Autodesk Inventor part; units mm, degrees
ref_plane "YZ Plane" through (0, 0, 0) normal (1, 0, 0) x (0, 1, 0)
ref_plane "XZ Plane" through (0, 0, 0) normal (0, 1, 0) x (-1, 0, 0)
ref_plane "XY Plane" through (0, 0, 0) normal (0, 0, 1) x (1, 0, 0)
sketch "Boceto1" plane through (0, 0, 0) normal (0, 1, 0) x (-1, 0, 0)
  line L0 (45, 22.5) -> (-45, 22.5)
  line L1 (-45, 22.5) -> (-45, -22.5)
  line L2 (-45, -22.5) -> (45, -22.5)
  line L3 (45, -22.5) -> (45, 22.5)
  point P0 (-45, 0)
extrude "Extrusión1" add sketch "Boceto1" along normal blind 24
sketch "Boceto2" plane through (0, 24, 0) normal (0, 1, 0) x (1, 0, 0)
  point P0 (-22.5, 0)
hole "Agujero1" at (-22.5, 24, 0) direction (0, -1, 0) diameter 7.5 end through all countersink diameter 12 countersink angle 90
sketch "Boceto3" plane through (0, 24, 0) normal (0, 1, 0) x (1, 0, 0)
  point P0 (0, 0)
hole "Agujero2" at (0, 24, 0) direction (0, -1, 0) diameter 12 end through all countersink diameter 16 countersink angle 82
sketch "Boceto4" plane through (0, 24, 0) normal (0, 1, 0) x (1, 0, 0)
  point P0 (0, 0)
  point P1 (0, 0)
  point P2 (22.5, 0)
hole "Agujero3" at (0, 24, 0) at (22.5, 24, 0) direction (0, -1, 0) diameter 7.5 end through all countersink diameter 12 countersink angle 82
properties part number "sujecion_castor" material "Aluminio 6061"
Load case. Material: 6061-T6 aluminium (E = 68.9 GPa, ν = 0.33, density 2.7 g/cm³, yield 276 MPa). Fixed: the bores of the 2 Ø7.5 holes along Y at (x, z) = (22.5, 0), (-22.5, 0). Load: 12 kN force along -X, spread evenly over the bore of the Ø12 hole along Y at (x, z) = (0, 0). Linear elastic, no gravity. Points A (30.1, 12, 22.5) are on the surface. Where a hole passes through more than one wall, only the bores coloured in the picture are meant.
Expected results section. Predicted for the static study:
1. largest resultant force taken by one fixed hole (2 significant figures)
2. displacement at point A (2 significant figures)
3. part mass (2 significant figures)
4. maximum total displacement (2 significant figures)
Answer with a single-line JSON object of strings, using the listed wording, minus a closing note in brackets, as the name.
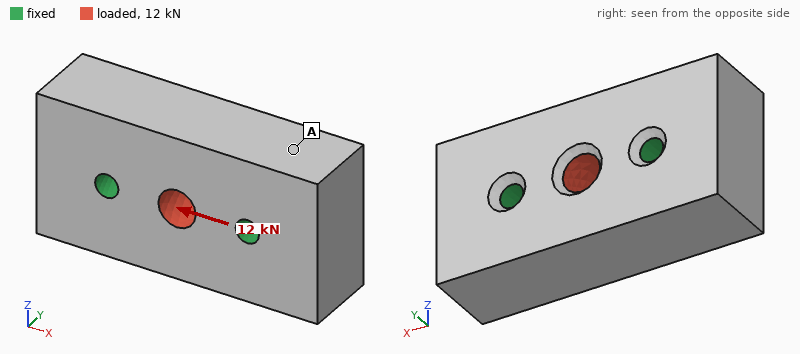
{"largest resultant force taken by one fixed hole": "6.0 kN", "displacement at point A": "1.4 µm", "part mass": "250 g", "maximum total displacement": "3.9 µm"}
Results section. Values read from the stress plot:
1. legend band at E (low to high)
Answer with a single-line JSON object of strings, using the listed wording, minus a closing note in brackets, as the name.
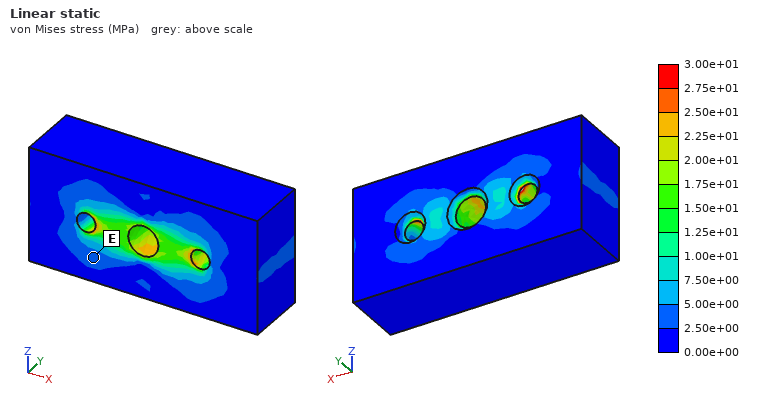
{"legend band at E": "2.50e+00 to 5.00e+00 MPa"}
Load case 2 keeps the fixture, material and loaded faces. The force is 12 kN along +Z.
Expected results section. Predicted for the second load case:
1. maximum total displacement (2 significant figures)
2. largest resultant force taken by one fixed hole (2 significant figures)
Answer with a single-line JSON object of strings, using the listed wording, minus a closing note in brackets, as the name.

{"maximum total displacement": "7.6 µm", "largest resultant force taken by one fixed hole": "6.0 kN"}
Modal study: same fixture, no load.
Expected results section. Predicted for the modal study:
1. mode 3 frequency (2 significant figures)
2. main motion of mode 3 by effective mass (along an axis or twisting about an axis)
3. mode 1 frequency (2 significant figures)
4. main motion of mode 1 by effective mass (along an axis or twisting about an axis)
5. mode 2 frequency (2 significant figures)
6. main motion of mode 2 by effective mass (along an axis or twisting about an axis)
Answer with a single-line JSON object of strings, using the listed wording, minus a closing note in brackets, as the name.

{"mode 3 frequency": "18 kHz", "main motion of mode 3 by effective mass": "twisting about Z", "mode 1 frequency": "15 kHz", "main motion of mode 1 by effective mass": "twisting about X", "mode 2 frequency": "16 kHz", "main motion of mode 2 by effective mass": "twisting about Y"}
